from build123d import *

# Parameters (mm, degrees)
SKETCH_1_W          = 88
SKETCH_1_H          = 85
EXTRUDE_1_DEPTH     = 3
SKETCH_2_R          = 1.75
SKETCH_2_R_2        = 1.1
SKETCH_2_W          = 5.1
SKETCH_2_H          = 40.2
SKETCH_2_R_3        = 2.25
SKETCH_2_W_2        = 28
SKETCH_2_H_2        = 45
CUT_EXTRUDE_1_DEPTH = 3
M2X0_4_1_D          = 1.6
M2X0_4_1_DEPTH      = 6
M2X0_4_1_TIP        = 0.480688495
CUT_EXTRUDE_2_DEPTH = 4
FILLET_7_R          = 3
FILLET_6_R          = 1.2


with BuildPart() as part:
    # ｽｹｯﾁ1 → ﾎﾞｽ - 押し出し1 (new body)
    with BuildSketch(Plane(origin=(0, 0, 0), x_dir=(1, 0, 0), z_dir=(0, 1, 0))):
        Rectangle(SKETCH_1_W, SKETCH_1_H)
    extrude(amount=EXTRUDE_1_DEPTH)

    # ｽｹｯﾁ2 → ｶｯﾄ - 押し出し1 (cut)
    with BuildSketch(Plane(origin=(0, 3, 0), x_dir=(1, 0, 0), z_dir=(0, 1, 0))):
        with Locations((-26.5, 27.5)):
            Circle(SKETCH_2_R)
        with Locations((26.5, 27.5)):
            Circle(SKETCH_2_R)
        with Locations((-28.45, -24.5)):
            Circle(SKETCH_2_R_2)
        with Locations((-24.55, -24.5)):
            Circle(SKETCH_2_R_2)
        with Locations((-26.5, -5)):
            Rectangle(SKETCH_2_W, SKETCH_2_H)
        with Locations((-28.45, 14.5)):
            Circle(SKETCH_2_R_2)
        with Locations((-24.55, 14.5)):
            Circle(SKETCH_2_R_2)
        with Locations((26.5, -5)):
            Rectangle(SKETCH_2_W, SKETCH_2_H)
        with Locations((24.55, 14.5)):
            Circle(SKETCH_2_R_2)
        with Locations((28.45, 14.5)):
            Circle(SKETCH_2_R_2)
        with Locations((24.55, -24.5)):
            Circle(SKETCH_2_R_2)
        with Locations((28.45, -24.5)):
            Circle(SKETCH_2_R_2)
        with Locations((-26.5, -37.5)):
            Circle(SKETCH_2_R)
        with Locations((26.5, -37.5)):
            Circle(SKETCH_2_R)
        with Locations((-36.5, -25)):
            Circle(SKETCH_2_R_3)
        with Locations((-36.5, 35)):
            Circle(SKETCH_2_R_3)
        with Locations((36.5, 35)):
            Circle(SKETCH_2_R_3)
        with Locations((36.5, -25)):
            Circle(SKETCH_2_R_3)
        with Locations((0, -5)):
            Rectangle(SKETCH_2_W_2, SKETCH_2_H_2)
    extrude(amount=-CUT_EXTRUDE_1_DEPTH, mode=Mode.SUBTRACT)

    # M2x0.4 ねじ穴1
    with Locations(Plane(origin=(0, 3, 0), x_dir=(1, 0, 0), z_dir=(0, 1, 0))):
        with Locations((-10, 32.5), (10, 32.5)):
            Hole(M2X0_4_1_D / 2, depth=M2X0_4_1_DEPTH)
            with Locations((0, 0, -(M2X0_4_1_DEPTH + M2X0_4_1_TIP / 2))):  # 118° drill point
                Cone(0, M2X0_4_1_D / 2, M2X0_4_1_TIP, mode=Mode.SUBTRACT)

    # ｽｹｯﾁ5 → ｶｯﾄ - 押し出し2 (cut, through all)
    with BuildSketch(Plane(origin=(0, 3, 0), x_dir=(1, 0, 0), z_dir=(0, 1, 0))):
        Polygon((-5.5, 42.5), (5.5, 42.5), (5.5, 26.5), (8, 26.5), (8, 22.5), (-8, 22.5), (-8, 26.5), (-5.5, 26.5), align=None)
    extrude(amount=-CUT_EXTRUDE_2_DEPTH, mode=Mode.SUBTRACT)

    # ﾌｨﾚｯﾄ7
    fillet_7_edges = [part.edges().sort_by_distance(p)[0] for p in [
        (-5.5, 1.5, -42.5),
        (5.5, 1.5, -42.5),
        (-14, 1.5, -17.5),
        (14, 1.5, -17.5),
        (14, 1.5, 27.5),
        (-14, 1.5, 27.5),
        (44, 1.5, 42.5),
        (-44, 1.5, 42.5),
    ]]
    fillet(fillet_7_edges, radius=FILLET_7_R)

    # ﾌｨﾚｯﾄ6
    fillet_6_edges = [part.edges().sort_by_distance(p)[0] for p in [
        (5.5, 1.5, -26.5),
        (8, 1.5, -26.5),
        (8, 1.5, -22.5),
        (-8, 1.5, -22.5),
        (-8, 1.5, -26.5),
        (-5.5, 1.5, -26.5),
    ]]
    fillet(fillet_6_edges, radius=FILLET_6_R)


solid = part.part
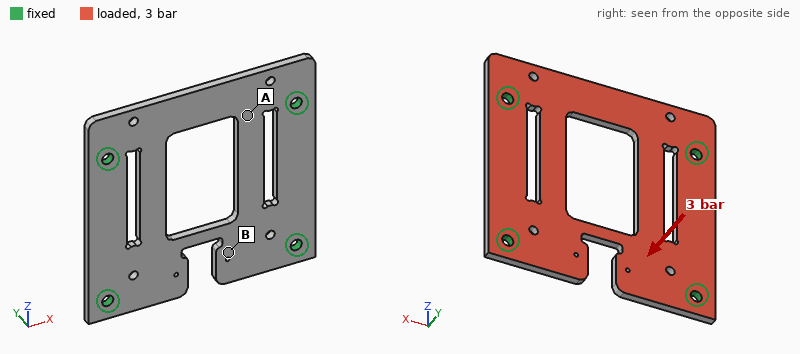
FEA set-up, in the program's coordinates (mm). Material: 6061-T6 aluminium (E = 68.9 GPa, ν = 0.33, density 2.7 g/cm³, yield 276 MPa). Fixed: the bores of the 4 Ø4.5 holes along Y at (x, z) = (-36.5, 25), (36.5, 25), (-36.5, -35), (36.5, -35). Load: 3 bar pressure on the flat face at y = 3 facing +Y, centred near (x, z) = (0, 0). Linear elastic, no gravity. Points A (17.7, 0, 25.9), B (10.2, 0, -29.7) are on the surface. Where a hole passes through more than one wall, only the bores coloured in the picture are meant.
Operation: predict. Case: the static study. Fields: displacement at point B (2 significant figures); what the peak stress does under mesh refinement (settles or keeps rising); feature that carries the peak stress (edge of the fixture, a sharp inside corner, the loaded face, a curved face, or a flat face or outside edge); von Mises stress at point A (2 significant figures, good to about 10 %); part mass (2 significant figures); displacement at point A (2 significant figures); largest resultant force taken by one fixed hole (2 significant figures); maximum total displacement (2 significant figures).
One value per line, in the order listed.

0.19 mm
keeps rising
edge of the fixture
43 MPa
44 g
0.14 mm
440 N
0.28 mm
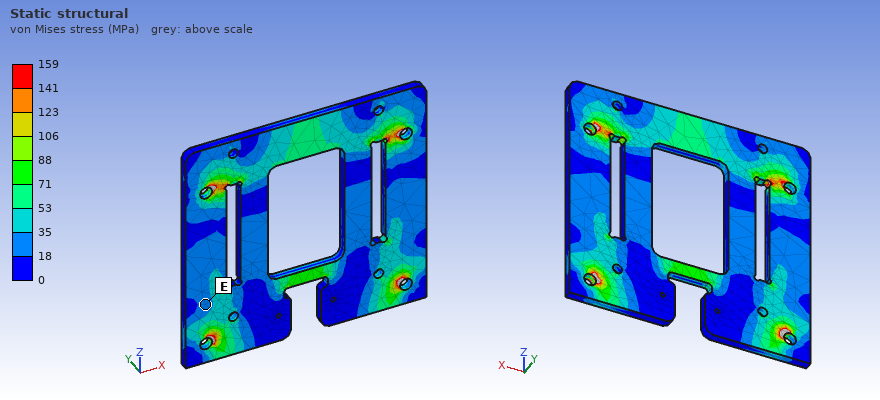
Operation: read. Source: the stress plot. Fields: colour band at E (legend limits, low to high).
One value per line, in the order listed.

18 to 35 MPa
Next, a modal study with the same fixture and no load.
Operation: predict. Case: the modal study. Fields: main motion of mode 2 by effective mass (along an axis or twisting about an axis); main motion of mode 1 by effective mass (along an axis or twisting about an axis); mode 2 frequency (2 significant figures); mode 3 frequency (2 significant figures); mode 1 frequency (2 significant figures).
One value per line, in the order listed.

twisting about X
along Y
2800 Hz
3700 Hz
2400 Hz
